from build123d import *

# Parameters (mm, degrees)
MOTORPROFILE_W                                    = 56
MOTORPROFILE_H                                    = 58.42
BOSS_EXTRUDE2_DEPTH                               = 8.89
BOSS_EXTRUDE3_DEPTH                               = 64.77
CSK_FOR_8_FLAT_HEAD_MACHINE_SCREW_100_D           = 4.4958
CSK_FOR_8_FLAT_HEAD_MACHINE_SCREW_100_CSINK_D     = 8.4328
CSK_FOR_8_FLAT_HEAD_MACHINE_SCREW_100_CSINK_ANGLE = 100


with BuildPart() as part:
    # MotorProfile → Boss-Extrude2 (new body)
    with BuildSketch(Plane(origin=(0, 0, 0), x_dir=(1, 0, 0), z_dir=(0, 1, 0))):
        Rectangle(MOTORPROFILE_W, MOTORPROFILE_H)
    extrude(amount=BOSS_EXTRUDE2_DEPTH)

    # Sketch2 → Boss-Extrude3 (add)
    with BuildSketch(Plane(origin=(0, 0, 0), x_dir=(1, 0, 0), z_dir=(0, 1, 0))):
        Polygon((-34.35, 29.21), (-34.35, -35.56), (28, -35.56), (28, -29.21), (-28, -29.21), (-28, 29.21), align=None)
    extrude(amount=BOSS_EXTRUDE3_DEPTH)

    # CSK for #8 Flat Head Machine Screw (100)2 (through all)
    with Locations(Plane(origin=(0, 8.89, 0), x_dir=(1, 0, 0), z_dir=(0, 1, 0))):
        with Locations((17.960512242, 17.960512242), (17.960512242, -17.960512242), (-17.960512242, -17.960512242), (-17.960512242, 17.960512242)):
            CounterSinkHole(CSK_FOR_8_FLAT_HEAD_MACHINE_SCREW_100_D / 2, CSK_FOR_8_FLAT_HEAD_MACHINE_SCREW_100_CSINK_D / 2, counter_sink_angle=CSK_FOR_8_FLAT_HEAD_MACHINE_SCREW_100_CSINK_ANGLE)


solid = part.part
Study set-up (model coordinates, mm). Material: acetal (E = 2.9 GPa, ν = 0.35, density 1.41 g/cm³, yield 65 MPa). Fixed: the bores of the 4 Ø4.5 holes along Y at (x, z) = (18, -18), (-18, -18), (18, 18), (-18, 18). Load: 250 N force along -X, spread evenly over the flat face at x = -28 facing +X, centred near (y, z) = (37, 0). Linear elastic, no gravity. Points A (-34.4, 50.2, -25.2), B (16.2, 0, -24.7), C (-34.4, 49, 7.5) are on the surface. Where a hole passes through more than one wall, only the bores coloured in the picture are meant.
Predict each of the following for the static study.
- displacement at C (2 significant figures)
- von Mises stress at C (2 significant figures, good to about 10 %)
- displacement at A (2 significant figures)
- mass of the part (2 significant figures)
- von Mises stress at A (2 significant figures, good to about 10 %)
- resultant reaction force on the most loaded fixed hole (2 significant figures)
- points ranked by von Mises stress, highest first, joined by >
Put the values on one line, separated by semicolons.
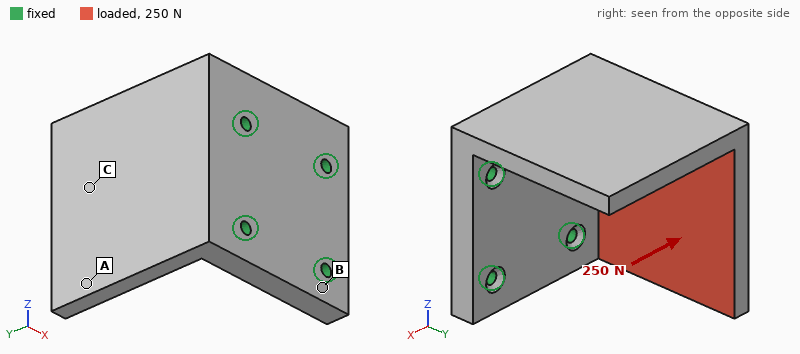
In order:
0.42 mm; 4.2 MPa; 0.80 mm; 110 g; 2.4 MPa; 190 N; C > A > B
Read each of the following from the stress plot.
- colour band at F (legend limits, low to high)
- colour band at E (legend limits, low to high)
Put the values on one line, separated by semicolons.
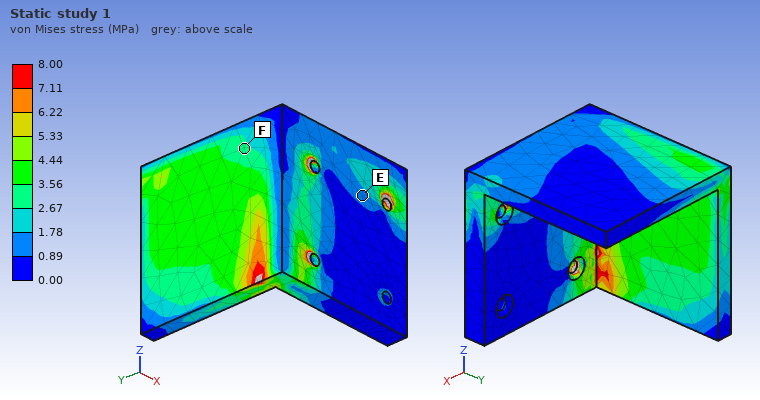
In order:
2.67 to 3.56 MPa; 0.89 to 1.78 MPa
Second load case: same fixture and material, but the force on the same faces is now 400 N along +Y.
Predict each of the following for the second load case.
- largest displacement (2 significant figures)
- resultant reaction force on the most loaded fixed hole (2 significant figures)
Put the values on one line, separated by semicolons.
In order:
99 µm; 230 N
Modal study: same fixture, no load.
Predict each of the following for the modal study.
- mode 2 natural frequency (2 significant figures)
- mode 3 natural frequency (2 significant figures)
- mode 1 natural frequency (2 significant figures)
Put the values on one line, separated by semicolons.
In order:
730 Hz; 990 Hz; 550 Hz
